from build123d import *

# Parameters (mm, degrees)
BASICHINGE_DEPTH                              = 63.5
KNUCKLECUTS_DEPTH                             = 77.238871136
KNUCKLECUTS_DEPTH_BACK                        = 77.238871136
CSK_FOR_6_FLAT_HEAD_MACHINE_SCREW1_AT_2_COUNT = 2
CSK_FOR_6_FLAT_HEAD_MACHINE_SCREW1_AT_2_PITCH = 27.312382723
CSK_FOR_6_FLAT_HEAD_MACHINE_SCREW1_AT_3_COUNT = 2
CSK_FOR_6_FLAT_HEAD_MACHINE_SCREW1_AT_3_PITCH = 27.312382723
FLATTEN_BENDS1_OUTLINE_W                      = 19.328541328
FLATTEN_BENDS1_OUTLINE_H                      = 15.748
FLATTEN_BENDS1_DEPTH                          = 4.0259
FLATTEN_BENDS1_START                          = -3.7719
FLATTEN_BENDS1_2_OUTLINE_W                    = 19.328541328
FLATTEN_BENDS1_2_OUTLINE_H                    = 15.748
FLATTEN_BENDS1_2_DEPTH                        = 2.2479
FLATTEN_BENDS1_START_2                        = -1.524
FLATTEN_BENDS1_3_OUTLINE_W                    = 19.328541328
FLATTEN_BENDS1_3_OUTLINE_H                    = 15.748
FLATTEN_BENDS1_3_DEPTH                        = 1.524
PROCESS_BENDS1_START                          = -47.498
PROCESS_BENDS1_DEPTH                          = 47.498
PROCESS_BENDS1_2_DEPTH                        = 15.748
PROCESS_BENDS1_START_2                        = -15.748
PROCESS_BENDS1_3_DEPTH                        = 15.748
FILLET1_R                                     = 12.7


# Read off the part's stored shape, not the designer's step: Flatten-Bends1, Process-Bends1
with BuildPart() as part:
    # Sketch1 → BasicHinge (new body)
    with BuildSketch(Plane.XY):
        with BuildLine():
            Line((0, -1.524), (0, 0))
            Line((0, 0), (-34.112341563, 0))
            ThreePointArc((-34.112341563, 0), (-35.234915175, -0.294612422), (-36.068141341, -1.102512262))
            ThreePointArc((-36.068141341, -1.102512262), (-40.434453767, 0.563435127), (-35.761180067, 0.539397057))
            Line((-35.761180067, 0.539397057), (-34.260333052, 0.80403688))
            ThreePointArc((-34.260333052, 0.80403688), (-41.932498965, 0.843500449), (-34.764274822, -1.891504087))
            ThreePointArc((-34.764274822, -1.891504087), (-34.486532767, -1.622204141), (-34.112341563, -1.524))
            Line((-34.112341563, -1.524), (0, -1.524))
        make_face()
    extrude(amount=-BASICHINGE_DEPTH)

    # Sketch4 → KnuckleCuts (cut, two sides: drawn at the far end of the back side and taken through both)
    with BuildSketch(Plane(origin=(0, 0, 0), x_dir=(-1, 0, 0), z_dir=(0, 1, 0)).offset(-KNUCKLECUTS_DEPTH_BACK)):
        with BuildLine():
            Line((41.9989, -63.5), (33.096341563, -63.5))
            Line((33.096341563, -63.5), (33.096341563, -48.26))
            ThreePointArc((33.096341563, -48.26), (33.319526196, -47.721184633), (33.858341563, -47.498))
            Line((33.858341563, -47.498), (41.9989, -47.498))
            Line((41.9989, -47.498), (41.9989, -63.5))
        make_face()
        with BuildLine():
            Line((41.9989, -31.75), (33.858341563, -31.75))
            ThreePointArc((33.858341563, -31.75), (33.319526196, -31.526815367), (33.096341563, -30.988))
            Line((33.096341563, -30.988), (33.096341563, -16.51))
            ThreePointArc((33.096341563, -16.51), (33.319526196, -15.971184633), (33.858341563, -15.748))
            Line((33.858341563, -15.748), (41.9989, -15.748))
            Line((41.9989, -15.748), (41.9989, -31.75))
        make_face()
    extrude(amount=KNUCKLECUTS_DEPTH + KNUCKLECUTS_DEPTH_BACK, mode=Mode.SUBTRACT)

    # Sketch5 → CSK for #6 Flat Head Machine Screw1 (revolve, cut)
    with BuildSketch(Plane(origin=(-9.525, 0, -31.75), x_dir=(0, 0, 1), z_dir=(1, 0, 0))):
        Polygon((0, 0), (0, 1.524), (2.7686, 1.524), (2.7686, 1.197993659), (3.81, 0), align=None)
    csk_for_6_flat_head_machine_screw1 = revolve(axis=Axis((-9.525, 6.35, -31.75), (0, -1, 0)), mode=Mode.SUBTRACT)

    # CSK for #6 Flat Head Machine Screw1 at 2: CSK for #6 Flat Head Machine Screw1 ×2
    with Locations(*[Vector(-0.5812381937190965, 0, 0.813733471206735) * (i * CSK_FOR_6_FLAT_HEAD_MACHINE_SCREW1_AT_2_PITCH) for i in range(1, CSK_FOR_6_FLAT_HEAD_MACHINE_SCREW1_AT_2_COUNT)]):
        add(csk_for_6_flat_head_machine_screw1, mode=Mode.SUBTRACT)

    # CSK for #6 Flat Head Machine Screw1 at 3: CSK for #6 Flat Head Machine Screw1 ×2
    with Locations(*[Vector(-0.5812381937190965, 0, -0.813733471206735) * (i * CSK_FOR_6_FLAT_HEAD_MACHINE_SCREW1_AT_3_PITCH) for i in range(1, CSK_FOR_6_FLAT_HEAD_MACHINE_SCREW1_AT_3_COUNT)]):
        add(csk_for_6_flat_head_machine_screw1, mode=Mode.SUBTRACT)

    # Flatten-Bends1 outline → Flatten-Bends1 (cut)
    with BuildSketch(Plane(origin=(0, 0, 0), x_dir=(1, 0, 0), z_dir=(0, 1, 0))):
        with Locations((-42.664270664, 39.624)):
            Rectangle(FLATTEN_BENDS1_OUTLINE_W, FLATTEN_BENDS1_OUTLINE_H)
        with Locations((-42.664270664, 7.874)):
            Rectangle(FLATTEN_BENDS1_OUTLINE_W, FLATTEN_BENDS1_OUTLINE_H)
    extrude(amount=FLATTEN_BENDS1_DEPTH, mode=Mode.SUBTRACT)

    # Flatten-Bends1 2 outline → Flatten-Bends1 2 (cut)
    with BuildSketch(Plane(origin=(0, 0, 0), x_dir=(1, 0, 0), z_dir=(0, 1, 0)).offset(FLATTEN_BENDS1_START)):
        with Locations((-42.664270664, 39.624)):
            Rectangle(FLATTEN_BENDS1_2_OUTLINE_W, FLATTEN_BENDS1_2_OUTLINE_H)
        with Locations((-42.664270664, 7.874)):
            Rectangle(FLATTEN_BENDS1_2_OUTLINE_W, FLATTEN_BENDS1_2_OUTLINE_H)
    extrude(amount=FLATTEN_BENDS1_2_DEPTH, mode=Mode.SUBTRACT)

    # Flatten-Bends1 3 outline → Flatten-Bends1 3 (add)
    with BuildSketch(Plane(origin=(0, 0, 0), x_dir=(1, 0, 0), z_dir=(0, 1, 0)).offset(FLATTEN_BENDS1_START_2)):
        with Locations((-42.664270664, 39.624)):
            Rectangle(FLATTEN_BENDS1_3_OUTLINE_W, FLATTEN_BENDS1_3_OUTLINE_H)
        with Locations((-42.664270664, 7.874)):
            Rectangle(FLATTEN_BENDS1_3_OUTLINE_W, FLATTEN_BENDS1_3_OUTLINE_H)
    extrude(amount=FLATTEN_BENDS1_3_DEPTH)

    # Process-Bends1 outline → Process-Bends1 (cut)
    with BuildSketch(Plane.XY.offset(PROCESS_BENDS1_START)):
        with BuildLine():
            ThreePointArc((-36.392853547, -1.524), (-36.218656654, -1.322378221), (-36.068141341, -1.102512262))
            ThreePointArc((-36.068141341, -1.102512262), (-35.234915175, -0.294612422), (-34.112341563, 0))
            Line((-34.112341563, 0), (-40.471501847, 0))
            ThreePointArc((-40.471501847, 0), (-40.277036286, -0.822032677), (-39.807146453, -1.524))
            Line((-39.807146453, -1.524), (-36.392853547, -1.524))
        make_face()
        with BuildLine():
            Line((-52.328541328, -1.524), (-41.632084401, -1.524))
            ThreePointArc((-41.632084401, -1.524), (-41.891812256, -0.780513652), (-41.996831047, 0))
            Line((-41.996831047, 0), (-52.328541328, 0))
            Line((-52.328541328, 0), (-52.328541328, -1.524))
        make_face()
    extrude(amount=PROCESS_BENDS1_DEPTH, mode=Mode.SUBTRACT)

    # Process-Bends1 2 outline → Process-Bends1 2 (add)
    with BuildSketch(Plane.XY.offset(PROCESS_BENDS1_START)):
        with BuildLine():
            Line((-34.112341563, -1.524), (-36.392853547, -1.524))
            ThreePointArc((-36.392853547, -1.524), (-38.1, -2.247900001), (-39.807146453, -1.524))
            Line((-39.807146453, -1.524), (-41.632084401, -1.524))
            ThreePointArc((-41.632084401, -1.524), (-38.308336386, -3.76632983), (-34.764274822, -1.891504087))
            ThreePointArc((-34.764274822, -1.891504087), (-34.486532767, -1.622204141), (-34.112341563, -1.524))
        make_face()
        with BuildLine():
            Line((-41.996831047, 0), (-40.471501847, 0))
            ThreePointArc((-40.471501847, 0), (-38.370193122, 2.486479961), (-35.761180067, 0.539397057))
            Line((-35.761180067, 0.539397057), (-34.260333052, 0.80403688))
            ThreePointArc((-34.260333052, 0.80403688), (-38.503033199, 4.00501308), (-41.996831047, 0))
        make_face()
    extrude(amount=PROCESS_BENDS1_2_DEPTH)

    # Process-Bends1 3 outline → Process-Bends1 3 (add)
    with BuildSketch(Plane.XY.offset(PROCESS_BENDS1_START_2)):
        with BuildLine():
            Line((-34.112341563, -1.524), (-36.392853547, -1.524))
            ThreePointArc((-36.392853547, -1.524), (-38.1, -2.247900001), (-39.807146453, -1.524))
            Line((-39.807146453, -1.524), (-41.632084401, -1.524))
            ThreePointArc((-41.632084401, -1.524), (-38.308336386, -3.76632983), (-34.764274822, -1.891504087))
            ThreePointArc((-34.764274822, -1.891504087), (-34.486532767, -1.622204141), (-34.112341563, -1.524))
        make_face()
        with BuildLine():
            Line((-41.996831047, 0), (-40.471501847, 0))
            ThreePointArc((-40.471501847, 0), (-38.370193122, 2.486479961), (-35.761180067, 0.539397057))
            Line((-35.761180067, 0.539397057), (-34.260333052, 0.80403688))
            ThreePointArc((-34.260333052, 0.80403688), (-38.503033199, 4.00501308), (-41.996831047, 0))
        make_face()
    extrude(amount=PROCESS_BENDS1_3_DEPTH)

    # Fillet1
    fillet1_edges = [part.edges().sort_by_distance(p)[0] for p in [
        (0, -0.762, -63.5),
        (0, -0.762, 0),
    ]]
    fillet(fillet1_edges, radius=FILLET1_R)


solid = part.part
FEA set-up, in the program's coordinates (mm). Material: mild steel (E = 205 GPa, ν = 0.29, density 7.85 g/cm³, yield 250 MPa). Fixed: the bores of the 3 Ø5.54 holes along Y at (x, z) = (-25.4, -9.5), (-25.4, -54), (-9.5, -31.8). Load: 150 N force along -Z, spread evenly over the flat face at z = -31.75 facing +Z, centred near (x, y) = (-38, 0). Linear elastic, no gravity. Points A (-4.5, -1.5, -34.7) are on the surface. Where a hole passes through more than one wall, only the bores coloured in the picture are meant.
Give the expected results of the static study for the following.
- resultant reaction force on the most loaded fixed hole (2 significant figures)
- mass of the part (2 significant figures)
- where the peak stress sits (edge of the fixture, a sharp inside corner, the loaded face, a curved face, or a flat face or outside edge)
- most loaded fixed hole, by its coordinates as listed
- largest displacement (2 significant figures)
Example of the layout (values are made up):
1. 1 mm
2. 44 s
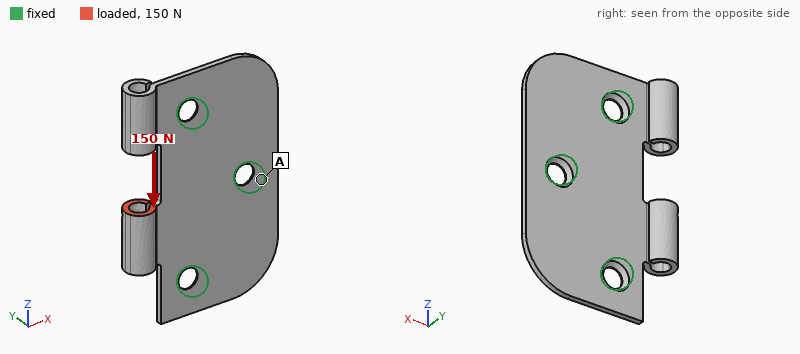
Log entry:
1. 110 N
2. 31 g
3. a curved face
4. (-25.4, -54)
5. 25 µm
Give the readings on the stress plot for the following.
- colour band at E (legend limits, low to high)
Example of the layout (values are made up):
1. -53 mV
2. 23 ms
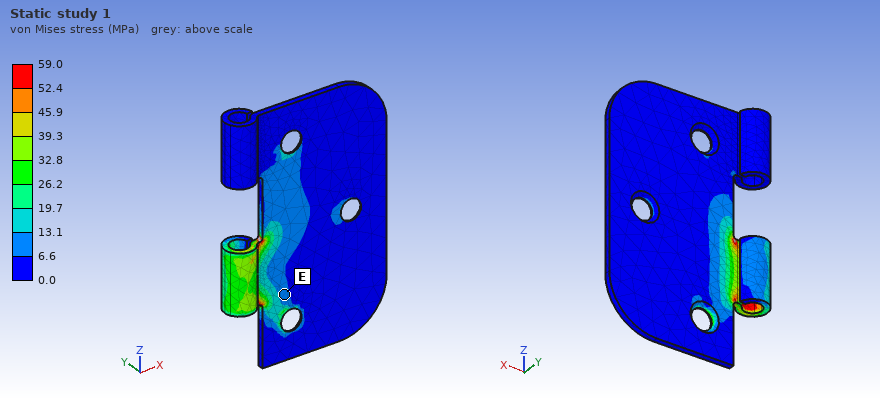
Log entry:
1. 6.6 to 13.1 MPa
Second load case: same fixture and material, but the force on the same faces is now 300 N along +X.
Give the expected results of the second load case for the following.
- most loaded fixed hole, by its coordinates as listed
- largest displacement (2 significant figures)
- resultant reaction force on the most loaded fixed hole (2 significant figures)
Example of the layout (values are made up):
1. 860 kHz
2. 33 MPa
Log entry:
1. (-9.5, -31.8)
2. 75 µm
3. 200 N
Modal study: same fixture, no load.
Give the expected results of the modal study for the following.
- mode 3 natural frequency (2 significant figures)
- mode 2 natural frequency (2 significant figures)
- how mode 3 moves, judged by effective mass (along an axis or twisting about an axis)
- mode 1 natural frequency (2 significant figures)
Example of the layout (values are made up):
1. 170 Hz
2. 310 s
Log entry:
1. 3400 Hz
2. 2800 Hz
3. twisting about X
4. 2300 Hz
